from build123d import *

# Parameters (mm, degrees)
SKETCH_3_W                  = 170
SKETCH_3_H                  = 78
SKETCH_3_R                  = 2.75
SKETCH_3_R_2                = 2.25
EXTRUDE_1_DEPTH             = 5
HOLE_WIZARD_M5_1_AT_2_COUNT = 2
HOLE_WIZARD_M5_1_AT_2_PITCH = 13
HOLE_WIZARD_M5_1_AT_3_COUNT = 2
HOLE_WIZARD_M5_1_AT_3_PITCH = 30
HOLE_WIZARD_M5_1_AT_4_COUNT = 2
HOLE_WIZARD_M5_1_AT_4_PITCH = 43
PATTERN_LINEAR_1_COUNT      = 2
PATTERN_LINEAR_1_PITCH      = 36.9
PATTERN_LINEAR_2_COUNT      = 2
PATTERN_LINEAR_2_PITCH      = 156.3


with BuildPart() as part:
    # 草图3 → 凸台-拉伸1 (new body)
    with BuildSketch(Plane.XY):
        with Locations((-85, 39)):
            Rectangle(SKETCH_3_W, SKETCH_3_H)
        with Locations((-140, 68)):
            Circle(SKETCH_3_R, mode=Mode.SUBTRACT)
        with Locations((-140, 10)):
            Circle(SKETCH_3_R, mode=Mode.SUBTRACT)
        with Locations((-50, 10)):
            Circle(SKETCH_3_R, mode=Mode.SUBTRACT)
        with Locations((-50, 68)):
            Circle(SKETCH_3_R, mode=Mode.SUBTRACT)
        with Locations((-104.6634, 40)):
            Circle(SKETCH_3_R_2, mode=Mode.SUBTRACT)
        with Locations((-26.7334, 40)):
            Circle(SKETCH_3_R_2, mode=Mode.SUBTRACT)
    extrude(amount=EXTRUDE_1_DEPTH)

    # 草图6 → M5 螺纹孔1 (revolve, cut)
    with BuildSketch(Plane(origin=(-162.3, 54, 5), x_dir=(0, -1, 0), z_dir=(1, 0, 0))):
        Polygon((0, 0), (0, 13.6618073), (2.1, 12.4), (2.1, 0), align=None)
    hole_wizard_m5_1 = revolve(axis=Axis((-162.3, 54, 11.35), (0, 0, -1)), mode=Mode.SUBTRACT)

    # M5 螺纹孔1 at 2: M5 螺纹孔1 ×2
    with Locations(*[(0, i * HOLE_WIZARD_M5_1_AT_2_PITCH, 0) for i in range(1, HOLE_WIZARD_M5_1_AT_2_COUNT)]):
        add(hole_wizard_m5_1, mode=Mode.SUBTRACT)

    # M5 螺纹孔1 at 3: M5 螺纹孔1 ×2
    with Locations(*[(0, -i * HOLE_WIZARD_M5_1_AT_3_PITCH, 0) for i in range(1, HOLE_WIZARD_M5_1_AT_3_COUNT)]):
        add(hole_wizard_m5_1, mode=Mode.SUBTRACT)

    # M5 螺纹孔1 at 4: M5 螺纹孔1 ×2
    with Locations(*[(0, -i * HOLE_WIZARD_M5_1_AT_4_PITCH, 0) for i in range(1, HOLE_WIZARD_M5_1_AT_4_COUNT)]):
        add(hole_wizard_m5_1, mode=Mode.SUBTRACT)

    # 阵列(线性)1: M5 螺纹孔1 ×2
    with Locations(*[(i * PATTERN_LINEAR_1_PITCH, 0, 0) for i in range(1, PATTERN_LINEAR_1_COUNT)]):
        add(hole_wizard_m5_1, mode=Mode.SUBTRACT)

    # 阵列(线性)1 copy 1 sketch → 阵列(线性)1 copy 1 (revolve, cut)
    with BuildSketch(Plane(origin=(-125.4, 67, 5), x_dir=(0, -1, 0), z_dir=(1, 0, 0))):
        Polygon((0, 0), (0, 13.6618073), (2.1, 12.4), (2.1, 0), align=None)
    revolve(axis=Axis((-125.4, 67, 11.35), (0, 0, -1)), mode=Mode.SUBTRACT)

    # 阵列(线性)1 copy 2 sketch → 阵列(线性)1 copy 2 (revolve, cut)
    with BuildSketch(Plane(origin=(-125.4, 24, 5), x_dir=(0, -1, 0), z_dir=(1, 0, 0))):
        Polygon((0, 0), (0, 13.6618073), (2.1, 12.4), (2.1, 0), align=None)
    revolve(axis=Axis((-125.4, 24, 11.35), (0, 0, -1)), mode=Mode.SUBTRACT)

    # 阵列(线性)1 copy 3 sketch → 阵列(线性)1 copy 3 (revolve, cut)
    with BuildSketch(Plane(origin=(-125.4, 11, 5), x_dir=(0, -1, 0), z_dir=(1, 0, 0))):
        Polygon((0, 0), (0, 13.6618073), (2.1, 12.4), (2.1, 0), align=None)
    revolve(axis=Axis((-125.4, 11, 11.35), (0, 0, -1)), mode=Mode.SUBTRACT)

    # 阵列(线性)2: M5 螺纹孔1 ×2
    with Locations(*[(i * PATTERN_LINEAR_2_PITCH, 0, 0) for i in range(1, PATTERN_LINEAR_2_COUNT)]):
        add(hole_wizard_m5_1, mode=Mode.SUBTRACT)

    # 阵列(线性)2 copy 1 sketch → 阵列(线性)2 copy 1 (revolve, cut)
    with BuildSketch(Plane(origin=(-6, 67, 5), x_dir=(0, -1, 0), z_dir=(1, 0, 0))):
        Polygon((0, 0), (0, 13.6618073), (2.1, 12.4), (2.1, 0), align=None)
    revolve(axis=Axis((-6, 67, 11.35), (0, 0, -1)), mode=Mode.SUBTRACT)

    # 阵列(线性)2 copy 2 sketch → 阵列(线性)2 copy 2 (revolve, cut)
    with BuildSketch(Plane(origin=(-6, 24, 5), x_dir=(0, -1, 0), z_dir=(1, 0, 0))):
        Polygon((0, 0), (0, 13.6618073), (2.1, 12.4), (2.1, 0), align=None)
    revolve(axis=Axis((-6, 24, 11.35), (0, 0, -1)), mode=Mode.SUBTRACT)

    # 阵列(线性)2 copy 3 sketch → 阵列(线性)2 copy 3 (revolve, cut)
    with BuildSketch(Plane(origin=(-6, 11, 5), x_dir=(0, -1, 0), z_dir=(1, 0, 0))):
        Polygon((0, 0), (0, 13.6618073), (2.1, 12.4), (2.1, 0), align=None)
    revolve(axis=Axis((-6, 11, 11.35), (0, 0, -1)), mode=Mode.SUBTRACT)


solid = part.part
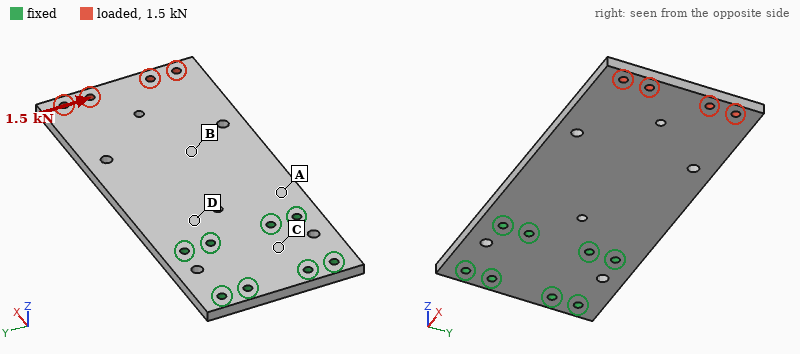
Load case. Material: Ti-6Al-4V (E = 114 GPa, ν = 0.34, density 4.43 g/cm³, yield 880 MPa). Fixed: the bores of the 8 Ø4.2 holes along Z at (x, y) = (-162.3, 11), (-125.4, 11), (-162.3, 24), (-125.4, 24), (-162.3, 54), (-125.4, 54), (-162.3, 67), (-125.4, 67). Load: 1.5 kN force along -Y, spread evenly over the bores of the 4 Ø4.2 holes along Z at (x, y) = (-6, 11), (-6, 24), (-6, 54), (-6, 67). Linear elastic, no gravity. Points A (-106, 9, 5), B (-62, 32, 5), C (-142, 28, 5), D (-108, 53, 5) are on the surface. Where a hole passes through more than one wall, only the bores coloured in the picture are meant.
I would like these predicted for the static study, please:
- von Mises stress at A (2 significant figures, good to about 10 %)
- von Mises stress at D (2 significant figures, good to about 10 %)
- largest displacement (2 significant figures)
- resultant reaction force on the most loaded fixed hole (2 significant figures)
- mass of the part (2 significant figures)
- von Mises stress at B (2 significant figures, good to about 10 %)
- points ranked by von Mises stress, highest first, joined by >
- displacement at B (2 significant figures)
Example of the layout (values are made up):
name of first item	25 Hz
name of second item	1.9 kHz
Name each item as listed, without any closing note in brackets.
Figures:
von Mises stress at A	24 MPa
von Mises stress at D	16 MPa
largest displacement	63 µm
resultant reaction force on the most loaded fixed hole	2.3 kN
mass of the part	290 g
von Mises stress at B	10 MPa
points ranked by von Mises stress, highest first, joined by >	A > D > B > C
displacement at B	22 µm
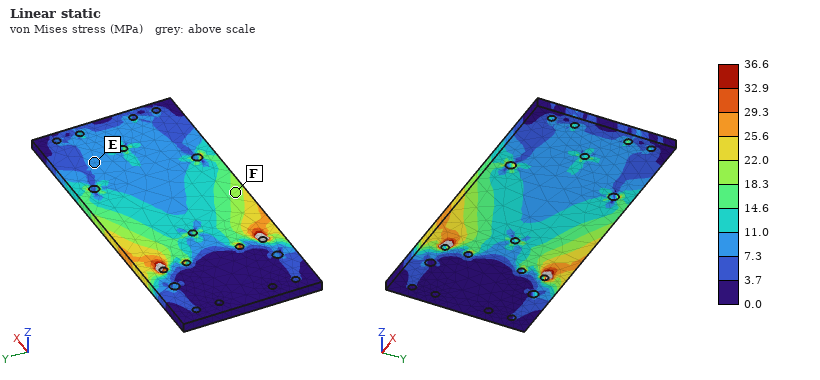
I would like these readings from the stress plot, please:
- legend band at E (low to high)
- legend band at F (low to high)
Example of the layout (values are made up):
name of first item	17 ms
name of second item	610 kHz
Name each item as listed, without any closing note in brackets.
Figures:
legend band at E	7.3 to 11.0 MPa
legend band at F	18.3 to 22.0 MPa
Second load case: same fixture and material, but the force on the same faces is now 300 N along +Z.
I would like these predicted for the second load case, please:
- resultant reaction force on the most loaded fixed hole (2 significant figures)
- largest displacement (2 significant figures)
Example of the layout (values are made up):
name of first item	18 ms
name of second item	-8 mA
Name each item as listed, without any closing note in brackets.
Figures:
resultant reaction force on the most loaded fixed hole	330 N
largest displacement	1.9 mm
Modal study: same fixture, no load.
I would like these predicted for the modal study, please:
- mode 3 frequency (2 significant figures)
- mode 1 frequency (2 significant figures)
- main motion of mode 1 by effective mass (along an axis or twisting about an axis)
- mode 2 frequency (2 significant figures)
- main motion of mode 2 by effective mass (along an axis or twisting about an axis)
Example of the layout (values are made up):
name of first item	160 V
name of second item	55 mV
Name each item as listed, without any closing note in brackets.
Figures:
mode 3 frequency	1600 Hz
mode 1 frequency	270 Hz
main motion of mode 1 by effective mass	along Z
mode 2 frequency	930 Hz
main motion of mode 2 by effective mass	twisting about X
